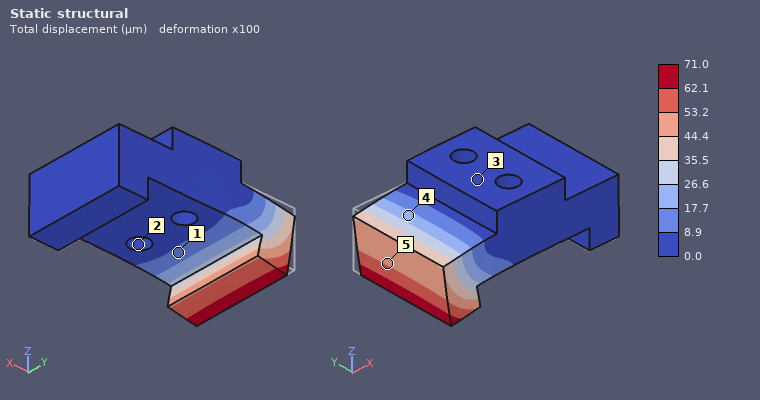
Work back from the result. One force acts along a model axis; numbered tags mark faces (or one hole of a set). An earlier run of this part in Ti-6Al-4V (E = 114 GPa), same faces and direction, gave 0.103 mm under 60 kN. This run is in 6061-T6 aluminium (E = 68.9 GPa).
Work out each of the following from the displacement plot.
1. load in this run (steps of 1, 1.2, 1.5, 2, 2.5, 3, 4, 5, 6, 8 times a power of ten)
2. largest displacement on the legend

25 kN
71.0 µm
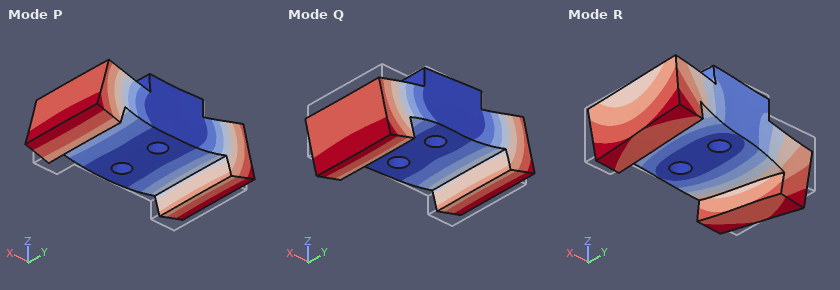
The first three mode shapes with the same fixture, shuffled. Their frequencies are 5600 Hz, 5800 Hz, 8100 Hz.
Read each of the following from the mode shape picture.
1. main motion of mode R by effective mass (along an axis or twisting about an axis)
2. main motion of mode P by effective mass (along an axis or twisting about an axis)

twisting about Z
along Z
